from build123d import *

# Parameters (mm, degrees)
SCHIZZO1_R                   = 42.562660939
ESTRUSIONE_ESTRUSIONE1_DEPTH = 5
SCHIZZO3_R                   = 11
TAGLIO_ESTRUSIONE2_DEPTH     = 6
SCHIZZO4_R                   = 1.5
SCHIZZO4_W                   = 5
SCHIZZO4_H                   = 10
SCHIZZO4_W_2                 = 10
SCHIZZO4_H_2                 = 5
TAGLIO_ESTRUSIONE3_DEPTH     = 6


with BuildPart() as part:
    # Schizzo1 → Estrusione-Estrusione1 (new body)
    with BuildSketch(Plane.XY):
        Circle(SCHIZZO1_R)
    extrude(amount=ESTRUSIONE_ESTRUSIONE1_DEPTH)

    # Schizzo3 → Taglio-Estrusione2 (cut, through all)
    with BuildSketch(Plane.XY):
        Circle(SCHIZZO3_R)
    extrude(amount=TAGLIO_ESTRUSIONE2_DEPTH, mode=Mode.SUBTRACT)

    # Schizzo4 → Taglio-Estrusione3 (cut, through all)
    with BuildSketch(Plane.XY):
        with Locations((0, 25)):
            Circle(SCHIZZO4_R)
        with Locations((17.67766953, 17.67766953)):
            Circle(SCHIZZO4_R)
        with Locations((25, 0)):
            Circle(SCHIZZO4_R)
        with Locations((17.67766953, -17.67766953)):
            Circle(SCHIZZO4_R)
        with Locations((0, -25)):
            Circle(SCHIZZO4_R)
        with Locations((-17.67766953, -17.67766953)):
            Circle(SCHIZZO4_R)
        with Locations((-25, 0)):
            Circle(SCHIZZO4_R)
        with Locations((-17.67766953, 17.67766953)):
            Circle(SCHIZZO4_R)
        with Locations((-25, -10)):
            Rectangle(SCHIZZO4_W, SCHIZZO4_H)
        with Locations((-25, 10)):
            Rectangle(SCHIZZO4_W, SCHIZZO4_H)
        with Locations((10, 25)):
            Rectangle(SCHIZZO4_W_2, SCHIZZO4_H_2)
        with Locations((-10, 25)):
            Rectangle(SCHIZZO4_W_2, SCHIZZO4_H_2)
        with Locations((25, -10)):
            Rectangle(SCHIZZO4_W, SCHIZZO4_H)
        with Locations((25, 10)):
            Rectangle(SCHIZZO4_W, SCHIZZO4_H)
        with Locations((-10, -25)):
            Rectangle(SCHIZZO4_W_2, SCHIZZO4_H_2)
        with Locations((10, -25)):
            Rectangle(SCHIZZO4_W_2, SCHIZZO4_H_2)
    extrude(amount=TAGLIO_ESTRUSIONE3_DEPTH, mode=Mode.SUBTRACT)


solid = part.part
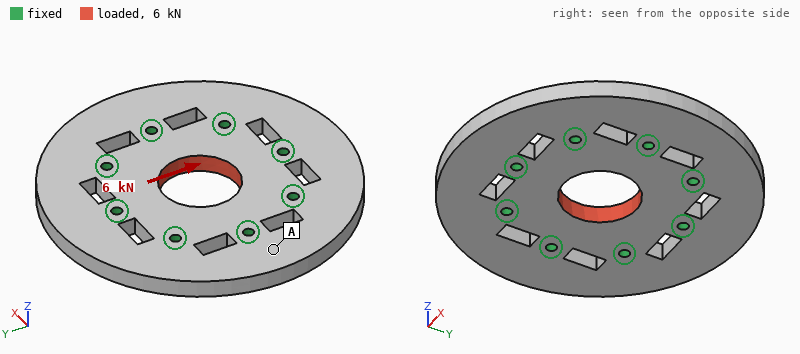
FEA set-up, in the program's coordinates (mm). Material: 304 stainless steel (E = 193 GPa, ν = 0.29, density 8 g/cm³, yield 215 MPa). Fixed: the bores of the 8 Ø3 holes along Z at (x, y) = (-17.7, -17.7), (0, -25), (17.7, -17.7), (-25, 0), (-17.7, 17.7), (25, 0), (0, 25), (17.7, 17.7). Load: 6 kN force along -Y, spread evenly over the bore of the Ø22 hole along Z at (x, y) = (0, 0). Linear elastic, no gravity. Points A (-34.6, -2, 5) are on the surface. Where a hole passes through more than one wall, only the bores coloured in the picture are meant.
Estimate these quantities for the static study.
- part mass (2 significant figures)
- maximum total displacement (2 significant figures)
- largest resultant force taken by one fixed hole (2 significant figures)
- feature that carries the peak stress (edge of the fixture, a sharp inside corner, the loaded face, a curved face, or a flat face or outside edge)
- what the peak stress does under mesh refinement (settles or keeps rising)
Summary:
190 g
1.6 µm
1.1 kN
edge of the fixture
keeps rising
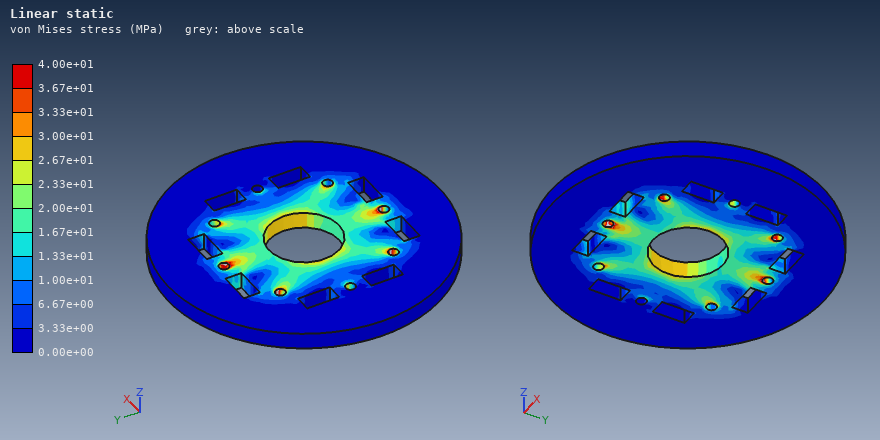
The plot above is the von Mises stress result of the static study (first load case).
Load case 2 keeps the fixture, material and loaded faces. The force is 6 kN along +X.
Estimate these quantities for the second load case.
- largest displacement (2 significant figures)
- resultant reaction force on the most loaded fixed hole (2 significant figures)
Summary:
1.6 µm
1.1 kN
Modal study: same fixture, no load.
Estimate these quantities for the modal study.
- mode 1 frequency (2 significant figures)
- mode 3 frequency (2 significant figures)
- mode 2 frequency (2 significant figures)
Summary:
8900 Hz
9100 Hz
9100 Hz
